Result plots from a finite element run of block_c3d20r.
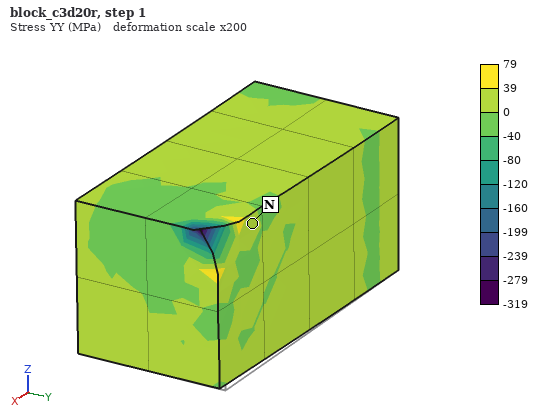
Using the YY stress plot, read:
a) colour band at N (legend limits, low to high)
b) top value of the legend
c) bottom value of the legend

0 to 39 MPa
79 MPa
-319 MPa
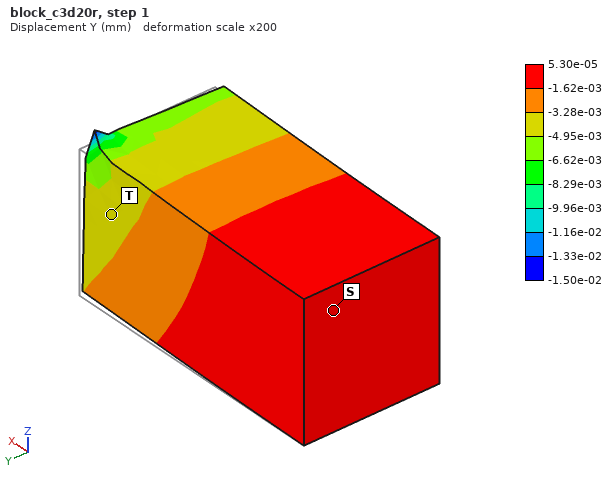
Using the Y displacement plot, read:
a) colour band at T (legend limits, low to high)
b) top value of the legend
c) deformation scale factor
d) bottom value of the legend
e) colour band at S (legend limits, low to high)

-4.95e-03 to -3.28e-03 mm
5.30e-05 mm
200
-1.50e-02 mm
-1.62e-03 to 5.30e-05 mm
